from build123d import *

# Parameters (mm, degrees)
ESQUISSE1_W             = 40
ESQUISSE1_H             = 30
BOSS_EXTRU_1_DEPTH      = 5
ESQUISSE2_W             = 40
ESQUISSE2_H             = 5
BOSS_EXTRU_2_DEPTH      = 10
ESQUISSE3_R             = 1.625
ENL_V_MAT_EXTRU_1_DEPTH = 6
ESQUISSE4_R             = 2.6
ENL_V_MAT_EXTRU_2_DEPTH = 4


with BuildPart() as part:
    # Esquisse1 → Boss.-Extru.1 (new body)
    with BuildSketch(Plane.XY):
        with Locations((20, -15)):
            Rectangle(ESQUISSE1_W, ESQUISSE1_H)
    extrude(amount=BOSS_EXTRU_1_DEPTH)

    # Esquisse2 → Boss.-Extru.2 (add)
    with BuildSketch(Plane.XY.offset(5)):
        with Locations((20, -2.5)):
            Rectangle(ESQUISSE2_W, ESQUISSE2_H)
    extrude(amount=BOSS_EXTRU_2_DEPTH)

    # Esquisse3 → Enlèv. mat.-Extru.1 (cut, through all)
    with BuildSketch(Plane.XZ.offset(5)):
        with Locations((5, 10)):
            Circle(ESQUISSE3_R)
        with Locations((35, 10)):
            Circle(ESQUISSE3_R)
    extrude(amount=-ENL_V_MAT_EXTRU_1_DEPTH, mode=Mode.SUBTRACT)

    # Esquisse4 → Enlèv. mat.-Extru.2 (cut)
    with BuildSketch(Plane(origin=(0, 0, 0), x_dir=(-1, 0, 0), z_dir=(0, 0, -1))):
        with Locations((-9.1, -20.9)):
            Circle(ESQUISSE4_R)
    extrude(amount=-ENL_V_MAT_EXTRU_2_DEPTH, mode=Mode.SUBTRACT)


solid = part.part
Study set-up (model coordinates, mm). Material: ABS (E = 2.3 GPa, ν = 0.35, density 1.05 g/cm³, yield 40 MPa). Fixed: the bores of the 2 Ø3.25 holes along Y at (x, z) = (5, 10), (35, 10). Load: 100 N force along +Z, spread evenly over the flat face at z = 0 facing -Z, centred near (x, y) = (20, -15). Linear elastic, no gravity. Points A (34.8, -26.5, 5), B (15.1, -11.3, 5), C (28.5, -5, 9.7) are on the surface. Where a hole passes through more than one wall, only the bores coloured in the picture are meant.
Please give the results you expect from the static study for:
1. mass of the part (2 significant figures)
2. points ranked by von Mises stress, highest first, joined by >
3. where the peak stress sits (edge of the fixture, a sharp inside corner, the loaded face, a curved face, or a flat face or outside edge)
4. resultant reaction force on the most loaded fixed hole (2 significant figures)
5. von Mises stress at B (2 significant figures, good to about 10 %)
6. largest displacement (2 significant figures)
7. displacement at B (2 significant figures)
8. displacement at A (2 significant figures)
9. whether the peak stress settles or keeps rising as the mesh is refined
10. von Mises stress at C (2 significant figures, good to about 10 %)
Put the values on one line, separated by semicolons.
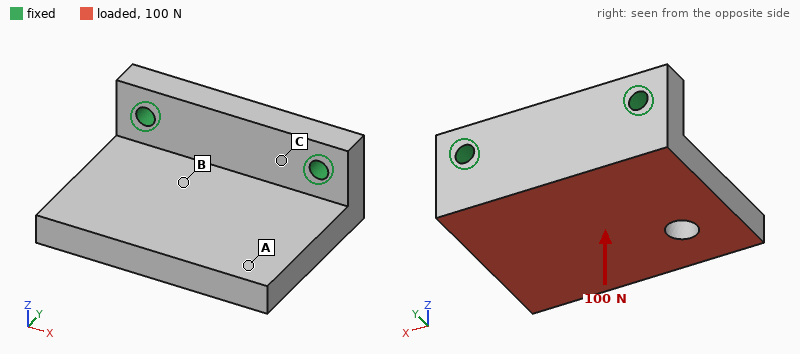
8.2 g; C > B > A; edge of the fixture; 54 N; 3.3 MPa; 0.54 mm; 0.14 mm; 0.45 mm; keeps rising; 4.6 MPa
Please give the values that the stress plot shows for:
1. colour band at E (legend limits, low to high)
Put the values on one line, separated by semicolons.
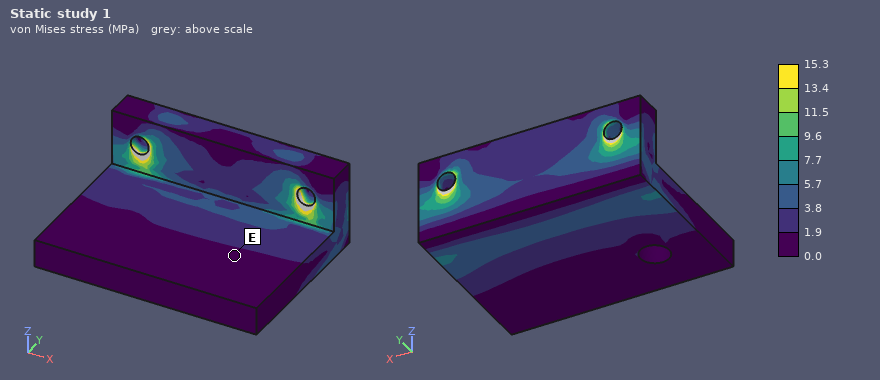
0.0 to 1.9 MPa
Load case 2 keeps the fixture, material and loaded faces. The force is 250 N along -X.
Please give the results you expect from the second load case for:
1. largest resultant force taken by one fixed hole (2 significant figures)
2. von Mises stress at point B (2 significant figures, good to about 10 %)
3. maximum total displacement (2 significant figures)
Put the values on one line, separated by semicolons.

180 N; 1.8 MPa; 0.11 mm
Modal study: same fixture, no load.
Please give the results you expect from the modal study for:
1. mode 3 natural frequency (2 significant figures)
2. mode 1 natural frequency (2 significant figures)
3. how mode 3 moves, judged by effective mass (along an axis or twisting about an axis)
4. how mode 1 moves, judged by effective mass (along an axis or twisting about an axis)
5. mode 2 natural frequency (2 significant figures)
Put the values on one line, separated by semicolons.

3600 Hz; 1100 Hz; along X; along Z; 2300 Hz
